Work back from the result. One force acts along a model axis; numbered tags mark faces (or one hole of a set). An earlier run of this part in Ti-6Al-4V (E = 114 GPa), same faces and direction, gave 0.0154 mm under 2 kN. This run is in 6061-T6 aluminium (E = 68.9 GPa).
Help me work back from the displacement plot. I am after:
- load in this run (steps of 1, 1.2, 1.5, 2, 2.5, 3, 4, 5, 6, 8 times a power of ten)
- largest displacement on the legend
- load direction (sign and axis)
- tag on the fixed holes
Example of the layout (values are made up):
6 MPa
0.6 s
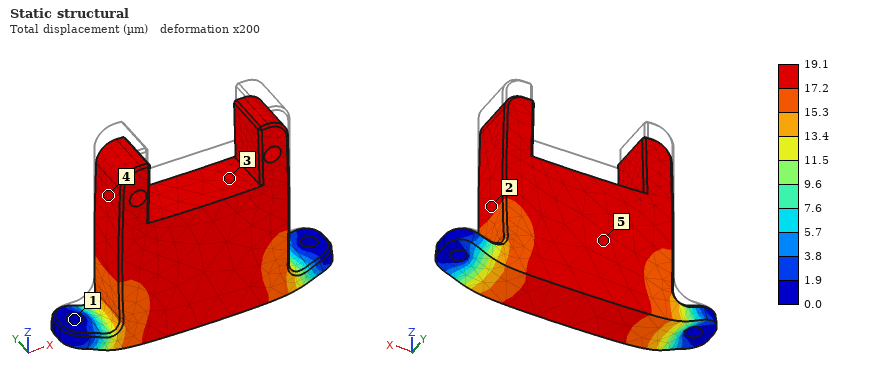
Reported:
1.5 kN
19.1 µm
-Z
1
